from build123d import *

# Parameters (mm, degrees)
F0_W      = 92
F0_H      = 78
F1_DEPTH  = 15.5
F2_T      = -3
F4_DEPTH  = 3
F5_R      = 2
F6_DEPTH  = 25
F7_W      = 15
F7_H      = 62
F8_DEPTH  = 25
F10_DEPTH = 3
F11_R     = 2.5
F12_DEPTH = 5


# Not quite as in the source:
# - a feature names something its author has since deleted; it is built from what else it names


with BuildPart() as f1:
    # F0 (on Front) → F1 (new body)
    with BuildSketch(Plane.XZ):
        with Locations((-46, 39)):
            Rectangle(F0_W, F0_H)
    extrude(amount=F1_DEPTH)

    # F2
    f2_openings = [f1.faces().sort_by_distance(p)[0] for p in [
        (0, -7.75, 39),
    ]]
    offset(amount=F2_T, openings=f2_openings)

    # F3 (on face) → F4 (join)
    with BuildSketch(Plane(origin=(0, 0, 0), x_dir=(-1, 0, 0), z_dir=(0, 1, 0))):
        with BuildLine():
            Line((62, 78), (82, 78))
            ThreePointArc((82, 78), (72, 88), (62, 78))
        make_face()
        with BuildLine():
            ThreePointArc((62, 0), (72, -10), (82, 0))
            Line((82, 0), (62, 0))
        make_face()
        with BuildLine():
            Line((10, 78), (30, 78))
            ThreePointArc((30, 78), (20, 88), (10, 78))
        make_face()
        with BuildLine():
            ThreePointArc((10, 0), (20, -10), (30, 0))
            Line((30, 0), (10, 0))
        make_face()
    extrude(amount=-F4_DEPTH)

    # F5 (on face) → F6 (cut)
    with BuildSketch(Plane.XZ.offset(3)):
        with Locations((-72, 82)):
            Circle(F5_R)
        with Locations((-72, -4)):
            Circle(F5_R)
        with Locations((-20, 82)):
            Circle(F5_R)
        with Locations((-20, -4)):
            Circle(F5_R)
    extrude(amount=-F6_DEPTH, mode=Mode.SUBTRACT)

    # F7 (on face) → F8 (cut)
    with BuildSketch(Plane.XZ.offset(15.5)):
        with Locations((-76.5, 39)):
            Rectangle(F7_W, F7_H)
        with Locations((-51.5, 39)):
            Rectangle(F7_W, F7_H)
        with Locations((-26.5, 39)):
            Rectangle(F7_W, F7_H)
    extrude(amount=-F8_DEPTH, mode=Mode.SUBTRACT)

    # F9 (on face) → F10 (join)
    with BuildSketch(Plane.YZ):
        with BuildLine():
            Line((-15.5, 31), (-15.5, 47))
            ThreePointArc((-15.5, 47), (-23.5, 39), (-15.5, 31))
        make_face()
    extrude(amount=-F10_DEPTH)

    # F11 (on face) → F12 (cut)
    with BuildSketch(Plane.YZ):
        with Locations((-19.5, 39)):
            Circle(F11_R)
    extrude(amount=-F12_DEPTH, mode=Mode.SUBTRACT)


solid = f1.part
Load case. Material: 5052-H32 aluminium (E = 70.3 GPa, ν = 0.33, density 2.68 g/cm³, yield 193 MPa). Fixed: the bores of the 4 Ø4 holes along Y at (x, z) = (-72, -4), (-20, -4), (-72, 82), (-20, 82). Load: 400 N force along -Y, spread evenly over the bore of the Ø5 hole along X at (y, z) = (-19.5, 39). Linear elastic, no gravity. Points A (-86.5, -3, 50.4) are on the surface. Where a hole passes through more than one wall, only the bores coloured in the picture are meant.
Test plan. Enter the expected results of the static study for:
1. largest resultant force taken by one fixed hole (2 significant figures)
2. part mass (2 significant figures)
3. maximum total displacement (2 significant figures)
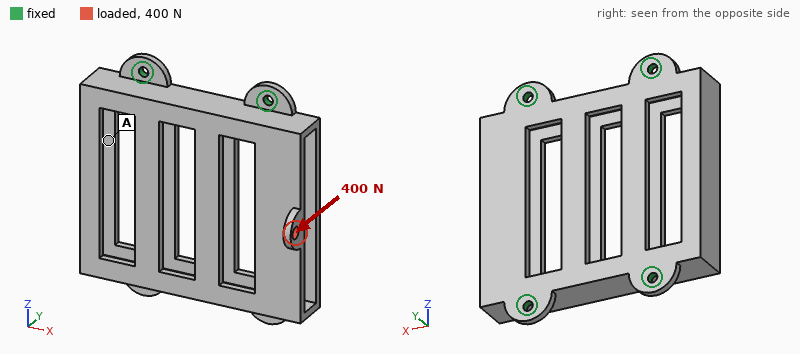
340 N
95 g
0.36 mm
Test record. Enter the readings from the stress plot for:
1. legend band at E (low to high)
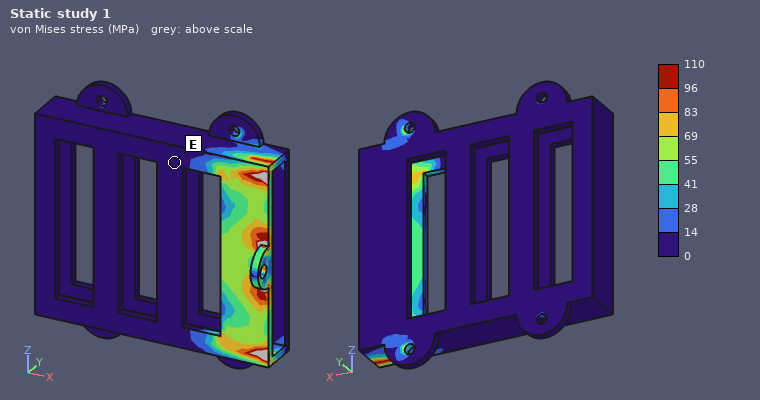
0 to 14 MPa
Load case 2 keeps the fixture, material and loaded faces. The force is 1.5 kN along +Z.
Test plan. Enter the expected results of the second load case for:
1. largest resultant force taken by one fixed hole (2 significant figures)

780 N
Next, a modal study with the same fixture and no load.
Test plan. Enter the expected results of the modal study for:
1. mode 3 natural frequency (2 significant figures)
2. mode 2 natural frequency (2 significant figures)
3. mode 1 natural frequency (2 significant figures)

2900 Hz
2600 Hz
2600 Hz
